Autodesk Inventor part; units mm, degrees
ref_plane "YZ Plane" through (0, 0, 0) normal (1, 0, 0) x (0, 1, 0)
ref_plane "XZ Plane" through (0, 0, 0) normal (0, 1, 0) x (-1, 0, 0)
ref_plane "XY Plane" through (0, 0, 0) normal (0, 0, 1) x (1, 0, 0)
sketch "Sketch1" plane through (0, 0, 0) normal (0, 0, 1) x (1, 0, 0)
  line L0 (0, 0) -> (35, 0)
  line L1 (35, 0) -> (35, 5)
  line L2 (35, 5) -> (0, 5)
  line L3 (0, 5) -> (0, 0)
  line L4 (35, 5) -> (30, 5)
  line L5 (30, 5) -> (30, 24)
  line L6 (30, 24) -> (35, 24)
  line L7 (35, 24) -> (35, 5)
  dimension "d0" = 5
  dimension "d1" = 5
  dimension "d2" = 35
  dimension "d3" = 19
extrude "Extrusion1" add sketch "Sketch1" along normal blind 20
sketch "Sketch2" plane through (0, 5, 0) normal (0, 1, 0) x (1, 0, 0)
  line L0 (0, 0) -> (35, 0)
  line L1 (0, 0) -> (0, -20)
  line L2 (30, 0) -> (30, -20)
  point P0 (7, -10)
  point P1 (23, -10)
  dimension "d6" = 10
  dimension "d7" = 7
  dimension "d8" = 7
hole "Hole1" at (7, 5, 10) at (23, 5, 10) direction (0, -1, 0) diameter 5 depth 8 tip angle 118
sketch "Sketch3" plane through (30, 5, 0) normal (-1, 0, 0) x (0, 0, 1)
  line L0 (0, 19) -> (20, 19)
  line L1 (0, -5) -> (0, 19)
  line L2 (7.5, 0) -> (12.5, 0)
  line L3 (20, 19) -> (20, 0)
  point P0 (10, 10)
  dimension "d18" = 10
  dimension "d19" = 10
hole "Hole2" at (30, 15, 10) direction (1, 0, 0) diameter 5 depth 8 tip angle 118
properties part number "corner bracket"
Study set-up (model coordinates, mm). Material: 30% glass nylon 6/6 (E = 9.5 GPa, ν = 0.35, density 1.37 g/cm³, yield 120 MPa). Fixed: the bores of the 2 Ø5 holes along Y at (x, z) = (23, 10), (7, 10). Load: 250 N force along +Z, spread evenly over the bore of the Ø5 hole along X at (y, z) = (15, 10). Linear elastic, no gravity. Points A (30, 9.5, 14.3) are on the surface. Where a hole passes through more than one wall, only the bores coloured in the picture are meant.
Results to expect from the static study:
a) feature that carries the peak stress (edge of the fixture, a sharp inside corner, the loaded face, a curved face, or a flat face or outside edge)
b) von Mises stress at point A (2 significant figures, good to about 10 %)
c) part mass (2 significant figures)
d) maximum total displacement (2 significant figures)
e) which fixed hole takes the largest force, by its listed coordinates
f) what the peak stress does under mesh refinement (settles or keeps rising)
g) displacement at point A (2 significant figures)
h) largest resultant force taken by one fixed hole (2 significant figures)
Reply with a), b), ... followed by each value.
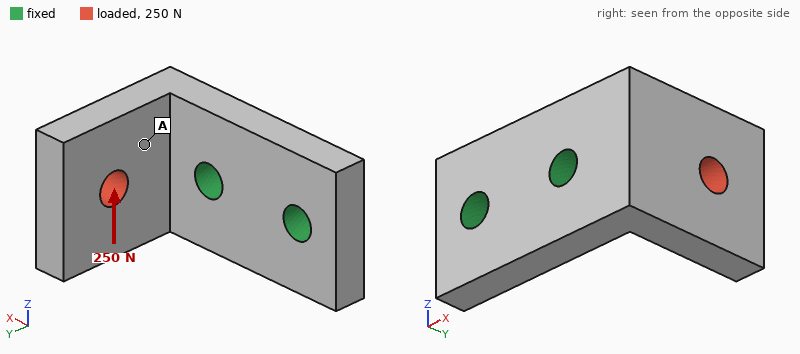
a) edge of the fixture
b) 9.5 MPa
c) 7.0 g
d) 0.21 mm
e) (23, 10)
f) keeps rising
g) 0.077 mm
h) 330 N
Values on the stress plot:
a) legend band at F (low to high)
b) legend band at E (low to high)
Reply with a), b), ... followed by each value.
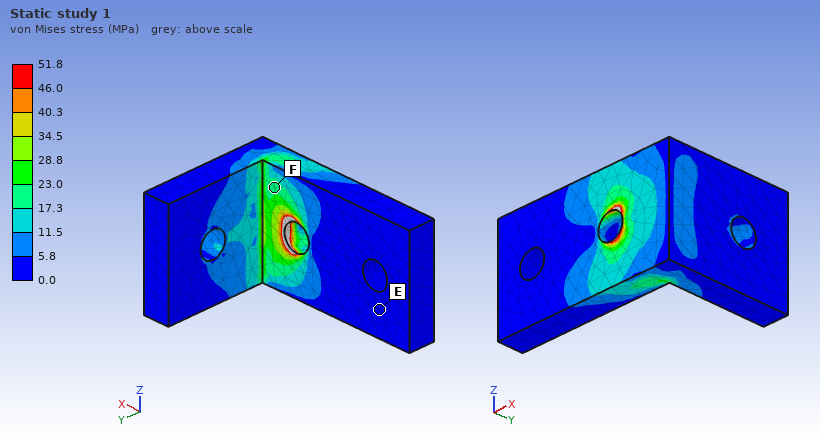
a) 17.3 to 23.0 MPa
b) 0.0 to 5.8 MPa
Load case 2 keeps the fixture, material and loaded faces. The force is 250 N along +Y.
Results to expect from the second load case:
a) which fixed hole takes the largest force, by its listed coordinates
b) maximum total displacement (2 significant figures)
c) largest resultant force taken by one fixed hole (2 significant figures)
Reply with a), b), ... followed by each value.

a) (23, 10)
b) 0.12 mm
c) 280 N
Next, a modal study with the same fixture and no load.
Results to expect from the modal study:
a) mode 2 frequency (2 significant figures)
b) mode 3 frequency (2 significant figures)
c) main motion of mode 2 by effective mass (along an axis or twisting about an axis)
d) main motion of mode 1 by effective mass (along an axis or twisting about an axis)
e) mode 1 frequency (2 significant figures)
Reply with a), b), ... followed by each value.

a) 4000 Hz
b) 8600 Hz
c) along Z
d) along X
e) 2900 Hz
